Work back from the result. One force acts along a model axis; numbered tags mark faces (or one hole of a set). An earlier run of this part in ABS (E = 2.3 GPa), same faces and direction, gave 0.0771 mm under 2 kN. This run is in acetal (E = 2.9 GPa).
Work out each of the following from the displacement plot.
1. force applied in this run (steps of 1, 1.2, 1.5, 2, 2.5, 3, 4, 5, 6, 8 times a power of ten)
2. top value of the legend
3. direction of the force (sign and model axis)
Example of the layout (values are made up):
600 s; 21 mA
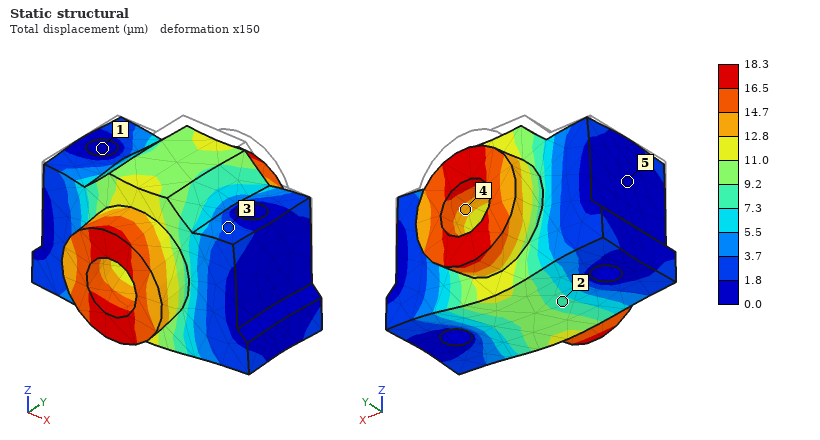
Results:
600 N; 18.3 µm; -Z
